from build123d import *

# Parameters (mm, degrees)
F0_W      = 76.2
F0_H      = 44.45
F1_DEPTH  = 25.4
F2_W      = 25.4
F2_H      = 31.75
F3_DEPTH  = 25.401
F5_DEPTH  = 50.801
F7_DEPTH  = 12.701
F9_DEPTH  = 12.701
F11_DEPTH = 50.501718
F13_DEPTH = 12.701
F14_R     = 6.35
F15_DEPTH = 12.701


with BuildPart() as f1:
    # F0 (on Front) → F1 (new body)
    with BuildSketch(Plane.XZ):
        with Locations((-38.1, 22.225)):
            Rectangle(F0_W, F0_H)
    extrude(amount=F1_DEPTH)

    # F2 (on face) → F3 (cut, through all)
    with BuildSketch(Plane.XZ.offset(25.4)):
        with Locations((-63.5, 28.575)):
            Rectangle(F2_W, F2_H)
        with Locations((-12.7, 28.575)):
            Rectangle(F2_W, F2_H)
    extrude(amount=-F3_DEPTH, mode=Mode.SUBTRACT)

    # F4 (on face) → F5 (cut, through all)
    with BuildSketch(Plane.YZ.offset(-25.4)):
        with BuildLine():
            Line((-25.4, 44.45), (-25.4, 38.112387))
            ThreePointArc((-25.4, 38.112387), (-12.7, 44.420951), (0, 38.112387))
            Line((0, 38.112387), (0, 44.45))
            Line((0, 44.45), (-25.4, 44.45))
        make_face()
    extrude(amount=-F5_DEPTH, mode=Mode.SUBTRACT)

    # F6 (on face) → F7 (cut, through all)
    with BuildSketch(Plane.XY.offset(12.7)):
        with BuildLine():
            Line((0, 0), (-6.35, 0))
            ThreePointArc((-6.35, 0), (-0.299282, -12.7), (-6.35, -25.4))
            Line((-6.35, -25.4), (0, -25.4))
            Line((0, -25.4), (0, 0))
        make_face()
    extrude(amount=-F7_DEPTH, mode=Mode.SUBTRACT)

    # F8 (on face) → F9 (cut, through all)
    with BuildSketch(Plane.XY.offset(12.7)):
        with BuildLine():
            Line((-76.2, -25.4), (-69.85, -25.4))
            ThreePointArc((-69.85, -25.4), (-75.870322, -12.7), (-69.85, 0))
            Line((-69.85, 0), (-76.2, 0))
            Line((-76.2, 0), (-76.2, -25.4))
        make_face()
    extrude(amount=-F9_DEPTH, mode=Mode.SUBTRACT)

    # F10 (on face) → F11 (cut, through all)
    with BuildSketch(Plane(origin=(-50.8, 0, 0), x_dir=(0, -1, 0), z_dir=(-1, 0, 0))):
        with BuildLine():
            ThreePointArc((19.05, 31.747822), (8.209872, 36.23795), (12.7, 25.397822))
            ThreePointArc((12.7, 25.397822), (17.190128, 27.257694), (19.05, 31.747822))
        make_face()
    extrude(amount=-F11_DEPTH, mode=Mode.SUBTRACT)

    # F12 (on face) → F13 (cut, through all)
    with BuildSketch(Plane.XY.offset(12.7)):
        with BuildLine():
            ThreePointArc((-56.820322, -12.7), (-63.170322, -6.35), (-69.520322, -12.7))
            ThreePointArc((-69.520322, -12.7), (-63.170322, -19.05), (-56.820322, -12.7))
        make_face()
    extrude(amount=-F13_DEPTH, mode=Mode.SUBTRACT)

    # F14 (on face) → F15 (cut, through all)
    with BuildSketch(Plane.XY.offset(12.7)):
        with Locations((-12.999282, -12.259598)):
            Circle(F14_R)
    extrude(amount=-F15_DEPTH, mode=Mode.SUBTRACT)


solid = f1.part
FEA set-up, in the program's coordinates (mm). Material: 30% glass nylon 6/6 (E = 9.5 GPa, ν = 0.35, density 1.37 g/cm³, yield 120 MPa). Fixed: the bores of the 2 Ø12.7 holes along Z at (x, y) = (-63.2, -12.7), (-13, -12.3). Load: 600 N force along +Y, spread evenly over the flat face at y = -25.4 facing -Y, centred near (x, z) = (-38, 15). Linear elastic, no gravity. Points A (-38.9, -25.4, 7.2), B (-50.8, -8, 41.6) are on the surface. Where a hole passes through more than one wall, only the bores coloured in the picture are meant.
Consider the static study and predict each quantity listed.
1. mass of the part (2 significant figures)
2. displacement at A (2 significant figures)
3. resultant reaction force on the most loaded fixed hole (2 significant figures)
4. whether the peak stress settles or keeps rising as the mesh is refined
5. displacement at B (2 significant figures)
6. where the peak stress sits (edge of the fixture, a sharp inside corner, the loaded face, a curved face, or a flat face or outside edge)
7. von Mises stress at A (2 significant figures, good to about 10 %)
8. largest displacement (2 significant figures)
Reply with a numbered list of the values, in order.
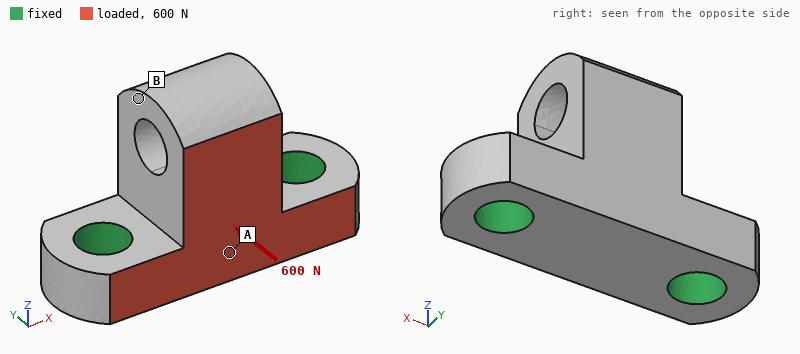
1. 49 g
2. 9.1 µm
3. 300 N
4. keeps rising
5. 31 µm
6. edge of the fixture
7. 1.3 MPa
8. 32 µm
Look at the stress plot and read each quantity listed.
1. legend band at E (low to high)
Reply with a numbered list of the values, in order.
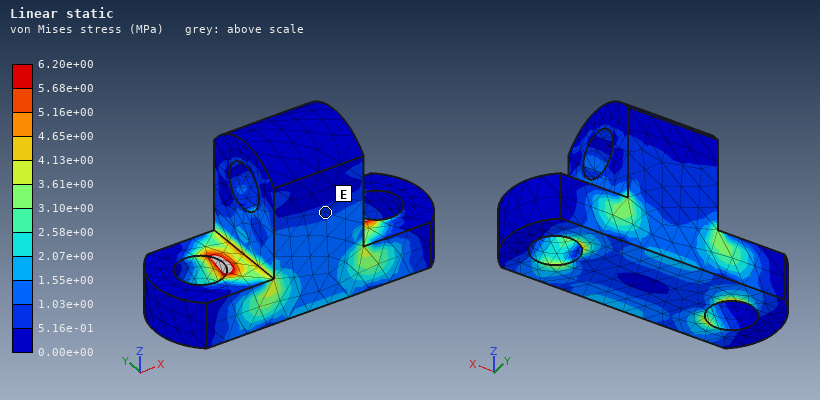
1. 5.16e-01 to 1.03e+00 MPa
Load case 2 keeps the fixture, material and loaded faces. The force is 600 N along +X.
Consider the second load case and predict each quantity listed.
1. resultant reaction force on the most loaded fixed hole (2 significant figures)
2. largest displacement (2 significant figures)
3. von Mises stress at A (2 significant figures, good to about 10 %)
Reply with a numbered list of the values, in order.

1. 360 N
2. 15 µm
3. 0.78 MPa
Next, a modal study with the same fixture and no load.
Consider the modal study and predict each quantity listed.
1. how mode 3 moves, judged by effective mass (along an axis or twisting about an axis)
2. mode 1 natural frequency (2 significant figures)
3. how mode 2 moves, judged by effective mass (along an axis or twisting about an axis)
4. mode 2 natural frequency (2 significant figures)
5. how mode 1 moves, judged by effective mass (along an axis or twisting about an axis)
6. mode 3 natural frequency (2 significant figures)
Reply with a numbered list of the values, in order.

1. along Z
2. 3500 Hz
3. along X
4. 6100 Hz
5. along Y
6. 8900 Hz
